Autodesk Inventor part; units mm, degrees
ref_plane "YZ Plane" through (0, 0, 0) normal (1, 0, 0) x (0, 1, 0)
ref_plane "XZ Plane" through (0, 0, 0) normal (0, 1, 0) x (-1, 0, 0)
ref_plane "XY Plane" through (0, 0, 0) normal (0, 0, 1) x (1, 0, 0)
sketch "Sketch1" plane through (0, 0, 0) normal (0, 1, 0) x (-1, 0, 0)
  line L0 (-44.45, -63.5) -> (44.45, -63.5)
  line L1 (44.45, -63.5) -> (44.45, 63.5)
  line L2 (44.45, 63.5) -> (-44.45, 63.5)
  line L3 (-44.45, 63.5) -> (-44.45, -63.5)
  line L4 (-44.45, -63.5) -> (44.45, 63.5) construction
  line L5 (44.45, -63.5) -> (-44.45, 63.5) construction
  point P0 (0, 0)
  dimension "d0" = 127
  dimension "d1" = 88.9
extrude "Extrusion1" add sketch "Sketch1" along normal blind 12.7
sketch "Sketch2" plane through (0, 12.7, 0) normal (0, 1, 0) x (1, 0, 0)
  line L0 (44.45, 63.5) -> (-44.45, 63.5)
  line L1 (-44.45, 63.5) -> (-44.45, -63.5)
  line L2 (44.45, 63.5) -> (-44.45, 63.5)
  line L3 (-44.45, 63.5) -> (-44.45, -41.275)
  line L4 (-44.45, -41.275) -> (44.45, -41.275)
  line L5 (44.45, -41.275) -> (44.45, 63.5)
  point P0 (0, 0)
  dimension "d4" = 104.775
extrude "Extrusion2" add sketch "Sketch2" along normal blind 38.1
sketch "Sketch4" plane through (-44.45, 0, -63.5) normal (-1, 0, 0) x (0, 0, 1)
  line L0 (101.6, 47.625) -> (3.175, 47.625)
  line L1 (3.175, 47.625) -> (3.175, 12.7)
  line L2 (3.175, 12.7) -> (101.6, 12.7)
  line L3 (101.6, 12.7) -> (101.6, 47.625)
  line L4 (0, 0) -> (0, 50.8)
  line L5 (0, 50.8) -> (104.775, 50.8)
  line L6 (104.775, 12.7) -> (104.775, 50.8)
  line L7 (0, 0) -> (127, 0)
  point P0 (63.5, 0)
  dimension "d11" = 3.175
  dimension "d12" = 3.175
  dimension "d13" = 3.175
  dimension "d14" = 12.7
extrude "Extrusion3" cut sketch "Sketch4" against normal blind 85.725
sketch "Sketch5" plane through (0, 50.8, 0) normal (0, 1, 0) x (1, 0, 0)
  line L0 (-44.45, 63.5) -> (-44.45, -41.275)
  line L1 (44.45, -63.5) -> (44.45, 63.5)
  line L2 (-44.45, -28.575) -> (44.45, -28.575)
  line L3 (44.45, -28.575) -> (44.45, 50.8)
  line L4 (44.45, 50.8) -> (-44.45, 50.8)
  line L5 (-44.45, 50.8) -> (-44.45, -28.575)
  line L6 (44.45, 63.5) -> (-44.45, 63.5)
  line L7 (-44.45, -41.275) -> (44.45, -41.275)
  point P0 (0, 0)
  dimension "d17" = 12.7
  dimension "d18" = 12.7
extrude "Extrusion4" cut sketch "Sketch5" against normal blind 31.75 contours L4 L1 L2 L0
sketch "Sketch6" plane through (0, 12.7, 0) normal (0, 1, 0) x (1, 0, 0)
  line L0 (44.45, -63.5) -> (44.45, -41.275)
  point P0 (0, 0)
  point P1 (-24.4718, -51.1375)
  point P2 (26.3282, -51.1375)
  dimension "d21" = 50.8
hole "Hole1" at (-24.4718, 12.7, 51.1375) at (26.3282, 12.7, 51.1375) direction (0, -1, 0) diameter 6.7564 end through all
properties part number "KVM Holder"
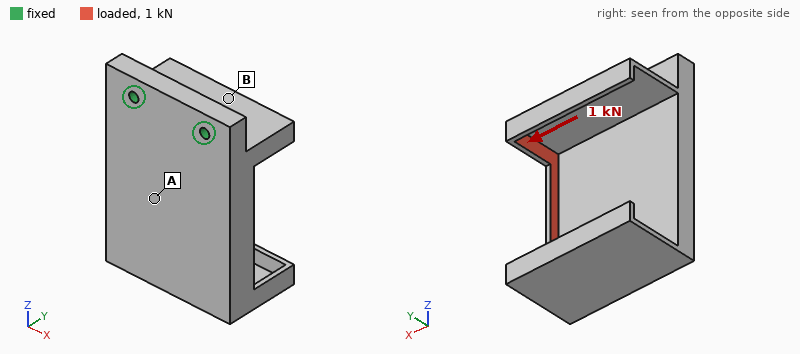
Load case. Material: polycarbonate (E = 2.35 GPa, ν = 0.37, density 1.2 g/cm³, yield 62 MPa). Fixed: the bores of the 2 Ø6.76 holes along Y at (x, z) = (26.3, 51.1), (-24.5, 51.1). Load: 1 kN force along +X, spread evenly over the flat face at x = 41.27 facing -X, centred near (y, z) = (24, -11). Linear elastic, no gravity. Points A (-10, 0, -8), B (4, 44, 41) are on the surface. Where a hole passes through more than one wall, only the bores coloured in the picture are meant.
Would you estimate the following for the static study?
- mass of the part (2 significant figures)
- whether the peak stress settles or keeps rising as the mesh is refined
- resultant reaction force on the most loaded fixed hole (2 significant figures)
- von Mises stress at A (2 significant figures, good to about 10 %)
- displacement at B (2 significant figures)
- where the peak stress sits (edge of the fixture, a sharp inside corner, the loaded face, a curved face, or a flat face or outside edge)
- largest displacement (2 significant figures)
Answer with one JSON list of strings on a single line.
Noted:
["210 g", "keeps rising", "1.3 kN", "2.1 MPa", "0.28 mm", "edge of the fixture", "1.6 mm"]
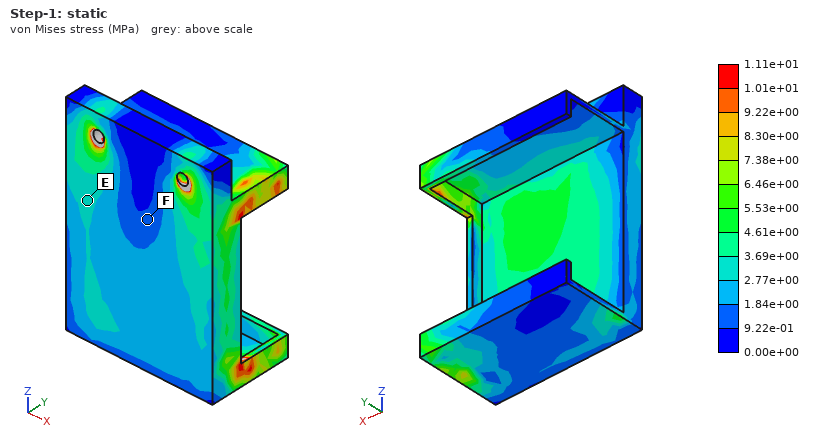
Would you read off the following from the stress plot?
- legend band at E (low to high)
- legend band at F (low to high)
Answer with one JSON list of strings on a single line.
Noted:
["2.77e+00 to 3.69e+00 MPa", "9.22e-01 to 1.84e+00 MPa"]
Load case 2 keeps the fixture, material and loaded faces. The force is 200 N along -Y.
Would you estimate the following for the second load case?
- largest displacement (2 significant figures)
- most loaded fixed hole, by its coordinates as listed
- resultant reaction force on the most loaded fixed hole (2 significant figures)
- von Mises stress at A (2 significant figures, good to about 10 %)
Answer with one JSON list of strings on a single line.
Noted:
["1.8 mm", "(26.3, 51.1)", "230 N", "2.0 MPa"]
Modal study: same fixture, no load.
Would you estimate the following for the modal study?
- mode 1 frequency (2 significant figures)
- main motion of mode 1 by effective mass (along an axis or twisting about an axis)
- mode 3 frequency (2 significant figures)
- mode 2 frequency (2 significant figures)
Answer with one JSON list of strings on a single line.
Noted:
["170 Hz", "along Y", "430 Hz", "410 Hz"]
